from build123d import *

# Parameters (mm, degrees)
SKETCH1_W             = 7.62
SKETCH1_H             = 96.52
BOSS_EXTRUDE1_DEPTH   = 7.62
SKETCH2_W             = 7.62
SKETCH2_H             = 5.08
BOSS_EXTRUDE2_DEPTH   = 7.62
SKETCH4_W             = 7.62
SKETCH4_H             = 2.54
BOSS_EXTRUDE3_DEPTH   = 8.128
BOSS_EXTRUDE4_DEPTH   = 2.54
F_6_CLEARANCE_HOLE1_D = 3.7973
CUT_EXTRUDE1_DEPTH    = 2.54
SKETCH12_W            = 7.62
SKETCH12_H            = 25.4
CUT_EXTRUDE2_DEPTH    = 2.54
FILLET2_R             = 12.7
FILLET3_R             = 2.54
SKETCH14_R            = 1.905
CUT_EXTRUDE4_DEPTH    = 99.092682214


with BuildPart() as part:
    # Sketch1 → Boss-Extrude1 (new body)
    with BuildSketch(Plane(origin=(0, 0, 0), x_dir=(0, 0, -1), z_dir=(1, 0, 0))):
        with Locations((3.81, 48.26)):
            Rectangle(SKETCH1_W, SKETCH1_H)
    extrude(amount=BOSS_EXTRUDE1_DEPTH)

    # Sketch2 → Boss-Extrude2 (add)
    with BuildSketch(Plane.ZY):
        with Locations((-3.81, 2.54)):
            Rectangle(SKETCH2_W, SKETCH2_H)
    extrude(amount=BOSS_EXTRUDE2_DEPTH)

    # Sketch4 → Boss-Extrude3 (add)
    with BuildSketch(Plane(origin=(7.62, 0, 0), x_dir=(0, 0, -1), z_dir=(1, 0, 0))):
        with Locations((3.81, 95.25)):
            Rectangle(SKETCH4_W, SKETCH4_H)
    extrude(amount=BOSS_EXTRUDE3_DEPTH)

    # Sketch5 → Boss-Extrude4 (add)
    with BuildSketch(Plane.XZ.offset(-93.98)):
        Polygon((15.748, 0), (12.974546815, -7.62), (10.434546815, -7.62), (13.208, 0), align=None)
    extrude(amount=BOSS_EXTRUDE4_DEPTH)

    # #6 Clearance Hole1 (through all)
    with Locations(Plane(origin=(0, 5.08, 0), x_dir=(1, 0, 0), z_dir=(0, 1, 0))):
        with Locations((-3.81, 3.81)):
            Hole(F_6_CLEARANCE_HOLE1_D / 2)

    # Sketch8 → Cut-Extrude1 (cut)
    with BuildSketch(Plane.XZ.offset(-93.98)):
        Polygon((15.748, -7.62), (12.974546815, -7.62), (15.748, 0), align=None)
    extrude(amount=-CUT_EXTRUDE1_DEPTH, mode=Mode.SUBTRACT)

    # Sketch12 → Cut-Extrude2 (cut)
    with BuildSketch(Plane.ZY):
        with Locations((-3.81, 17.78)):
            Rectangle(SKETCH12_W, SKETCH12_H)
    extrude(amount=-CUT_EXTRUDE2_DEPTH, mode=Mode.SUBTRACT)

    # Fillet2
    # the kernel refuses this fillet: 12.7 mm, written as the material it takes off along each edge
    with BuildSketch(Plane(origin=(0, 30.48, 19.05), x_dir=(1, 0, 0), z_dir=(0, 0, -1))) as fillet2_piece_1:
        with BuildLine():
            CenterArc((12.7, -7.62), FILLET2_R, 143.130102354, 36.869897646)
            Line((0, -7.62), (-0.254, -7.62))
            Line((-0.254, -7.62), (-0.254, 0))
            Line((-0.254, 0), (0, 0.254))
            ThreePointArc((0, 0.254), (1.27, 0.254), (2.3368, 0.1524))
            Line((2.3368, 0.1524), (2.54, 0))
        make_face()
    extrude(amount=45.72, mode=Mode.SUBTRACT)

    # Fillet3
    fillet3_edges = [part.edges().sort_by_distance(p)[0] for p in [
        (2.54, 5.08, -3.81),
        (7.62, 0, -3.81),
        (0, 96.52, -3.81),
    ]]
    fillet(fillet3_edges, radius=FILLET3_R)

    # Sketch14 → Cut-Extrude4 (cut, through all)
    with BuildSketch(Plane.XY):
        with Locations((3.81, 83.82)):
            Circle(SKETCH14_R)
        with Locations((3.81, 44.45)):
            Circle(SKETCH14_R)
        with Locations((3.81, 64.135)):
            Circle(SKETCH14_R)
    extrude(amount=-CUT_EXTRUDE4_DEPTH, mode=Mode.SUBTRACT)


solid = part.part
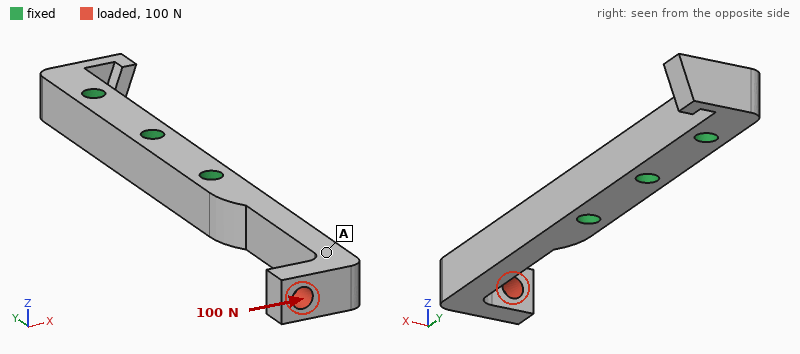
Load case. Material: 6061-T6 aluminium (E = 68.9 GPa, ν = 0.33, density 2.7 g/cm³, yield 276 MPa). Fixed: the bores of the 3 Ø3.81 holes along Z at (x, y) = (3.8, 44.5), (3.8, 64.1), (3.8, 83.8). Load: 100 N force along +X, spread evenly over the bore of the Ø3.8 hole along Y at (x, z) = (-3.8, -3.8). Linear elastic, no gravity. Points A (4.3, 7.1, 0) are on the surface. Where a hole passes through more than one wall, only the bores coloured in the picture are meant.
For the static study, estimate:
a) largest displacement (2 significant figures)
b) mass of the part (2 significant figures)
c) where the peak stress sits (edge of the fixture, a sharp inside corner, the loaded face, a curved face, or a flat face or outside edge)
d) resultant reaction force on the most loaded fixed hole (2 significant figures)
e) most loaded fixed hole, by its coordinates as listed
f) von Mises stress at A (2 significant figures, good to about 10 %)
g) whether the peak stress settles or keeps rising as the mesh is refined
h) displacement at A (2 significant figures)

0.30 mm
14 g
a sharp inside corner
140 N
(3.8, 44.5)
10 MPa
keeps rising
0.20 mm
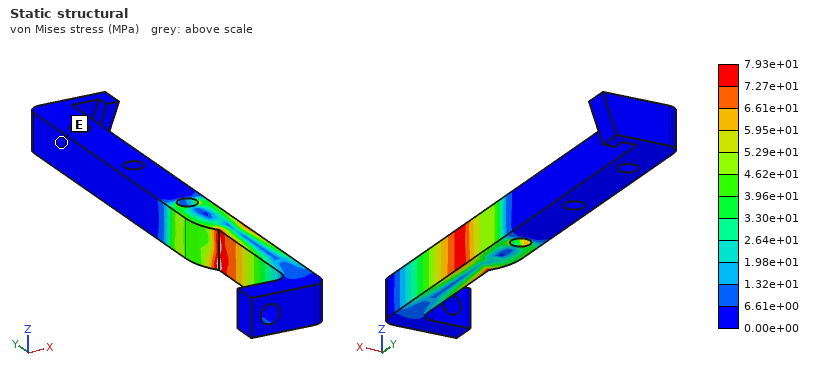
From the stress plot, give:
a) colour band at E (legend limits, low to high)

0.00e+00 to 6.61e+00 MPa
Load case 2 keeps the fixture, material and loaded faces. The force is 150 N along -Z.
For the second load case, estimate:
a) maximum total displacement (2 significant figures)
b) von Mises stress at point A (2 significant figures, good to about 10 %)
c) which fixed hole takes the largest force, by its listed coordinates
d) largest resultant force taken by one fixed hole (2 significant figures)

0.36 mm
44 MPa
(3.8, 44.5)
160 N
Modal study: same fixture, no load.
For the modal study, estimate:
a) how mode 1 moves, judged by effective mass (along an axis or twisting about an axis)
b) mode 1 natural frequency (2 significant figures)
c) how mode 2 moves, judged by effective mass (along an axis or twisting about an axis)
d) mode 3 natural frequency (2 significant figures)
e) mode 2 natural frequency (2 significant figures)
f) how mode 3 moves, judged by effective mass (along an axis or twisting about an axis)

along X
2200 Hz
along Z
8600 Hz
2700 Hz
twisting about Y
